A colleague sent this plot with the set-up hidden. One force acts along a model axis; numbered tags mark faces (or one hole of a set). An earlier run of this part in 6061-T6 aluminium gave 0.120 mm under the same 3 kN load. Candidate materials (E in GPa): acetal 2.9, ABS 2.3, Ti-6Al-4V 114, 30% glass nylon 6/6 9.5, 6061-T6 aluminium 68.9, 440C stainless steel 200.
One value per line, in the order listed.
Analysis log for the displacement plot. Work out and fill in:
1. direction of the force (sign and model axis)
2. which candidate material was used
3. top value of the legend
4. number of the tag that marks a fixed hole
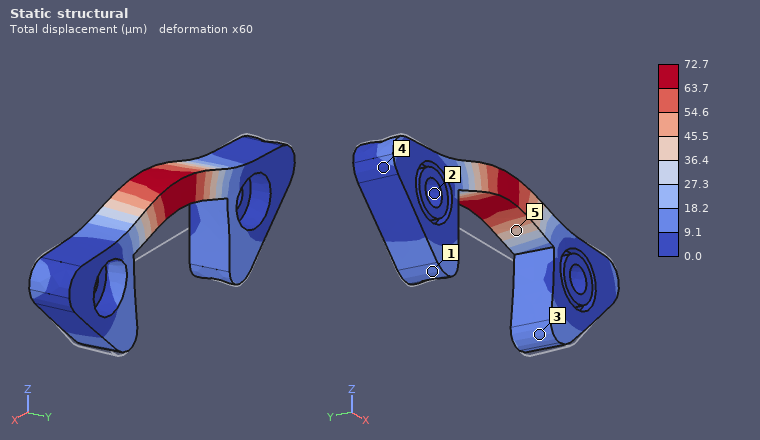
+Z
Ti-6Al-4V
72.7 µm
2
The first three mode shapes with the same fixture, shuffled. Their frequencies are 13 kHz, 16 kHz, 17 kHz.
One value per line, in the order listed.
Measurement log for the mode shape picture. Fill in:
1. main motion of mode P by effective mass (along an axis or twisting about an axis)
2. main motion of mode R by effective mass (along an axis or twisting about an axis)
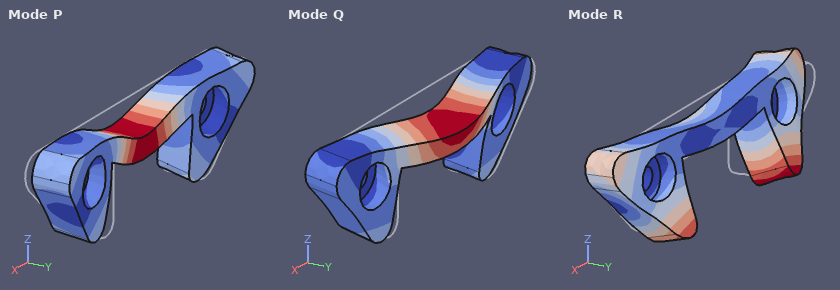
along Z
twisting about X
